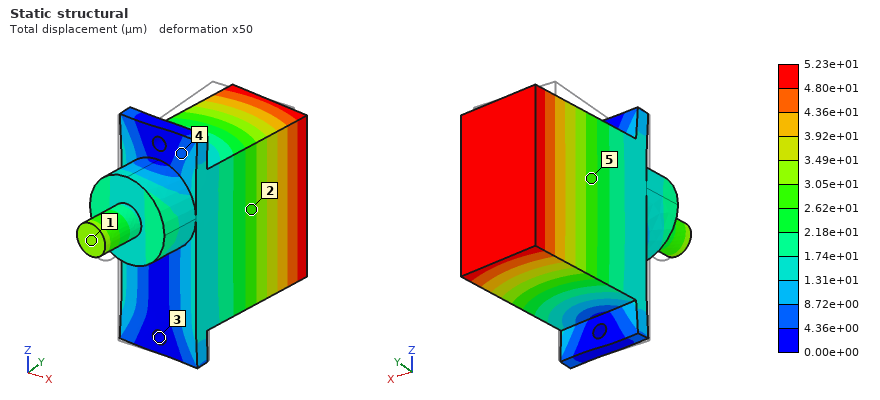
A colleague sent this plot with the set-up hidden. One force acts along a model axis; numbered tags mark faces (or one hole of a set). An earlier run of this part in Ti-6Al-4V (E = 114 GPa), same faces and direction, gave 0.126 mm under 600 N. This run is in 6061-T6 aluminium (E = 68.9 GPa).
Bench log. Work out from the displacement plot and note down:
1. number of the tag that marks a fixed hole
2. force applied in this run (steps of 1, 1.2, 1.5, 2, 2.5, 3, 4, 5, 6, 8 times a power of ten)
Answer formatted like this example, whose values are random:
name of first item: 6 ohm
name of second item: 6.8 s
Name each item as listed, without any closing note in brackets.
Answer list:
number of the tag that marks a fixed hole: 3
force applied in this run: 150 N
